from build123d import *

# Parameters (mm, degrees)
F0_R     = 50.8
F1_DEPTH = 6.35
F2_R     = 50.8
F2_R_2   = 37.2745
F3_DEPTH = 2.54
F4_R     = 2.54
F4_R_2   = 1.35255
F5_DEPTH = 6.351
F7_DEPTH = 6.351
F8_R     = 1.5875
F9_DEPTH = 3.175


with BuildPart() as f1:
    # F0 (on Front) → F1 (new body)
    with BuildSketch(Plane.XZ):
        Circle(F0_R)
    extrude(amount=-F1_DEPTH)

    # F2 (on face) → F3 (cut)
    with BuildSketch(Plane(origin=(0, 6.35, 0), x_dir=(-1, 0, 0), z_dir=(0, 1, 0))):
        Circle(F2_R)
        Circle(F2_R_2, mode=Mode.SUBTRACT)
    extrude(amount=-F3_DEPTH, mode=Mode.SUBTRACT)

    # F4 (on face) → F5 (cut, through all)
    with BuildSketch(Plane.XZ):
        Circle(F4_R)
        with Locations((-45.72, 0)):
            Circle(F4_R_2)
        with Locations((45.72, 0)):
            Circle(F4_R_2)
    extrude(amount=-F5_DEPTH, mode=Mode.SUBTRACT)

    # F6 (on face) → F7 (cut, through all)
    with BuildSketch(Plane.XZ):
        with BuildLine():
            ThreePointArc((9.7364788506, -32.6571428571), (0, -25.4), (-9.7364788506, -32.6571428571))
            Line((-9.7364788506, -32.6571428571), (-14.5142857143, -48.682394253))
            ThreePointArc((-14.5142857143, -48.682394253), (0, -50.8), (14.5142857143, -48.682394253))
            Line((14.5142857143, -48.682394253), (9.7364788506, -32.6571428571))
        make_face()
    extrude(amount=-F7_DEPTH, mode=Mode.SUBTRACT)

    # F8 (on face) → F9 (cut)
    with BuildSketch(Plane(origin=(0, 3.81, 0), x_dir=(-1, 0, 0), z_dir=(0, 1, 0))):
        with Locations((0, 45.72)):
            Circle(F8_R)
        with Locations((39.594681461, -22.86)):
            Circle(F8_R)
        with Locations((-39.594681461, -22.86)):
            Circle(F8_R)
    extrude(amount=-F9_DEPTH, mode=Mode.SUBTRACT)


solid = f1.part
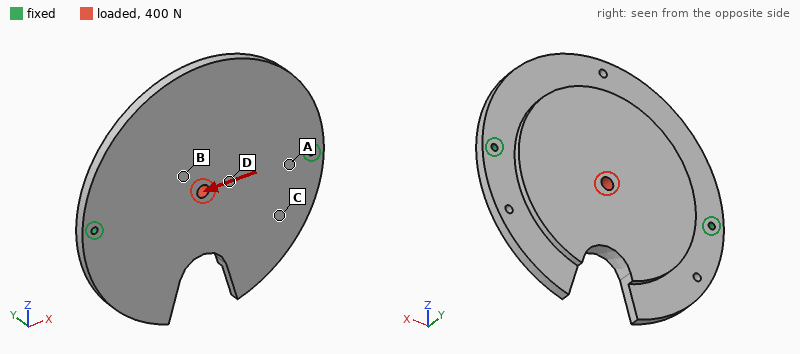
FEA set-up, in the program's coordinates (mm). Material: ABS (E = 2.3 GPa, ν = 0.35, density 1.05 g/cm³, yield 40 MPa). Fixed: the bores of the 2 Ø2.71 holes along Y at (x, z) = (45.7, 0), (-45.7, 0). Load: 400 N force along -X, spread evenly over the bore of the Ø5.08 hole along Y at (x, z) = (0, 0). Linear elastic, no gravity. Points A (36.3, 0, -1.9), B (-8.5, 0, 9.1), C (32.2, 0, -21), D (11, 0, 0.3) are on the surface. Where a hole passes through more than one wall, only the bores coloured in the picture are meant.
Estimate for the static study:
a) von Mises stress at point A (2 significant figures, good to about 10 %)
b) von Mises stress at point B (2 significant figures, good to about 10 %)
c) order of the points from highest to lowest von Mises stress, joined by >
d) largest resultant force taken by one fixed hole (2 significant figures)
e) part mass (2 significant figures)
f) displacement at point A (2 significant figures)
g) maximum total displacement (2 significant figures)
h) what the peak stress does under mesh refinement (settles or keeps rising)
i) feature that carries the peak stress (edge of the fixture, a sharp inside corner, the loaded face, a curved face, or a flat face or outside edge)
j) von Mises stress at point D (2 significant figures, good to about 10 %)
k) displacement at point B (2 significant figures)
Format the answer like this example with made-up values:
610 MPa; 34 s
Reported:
2.6 MPa; 0.99 MPa; A > D > B > C; 200 N; 41 g; 16 µm; 48 µm; keeps rising; edge of the fixture; 2.0 MPa; 35 µm
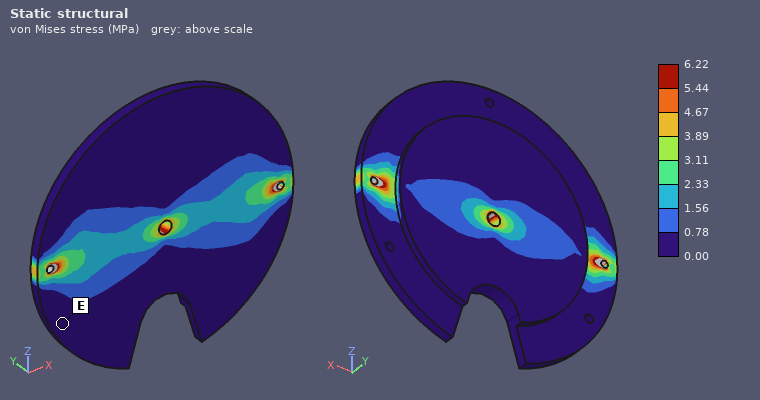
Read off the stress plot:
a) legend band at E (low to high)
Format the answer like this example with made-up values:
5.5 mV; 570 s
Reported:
0.00 to 0.78 MPa
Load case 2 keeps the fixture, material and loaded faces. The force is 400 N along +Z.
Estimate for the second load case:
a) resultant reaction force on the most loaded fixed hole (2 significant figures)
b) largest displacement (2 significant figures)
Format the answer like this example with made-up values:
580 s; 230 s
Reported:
200 N; 0.43 mm
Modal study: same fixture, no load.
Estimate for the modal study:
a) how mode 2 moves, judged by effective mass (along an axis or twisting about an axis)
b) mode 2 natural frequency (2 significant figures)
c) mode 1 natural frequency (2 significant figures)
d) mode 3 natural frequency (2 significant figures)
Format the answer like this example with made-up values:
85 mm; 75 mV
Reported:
along Y; 500 Hz; 270 Hz; 1000 Hz
